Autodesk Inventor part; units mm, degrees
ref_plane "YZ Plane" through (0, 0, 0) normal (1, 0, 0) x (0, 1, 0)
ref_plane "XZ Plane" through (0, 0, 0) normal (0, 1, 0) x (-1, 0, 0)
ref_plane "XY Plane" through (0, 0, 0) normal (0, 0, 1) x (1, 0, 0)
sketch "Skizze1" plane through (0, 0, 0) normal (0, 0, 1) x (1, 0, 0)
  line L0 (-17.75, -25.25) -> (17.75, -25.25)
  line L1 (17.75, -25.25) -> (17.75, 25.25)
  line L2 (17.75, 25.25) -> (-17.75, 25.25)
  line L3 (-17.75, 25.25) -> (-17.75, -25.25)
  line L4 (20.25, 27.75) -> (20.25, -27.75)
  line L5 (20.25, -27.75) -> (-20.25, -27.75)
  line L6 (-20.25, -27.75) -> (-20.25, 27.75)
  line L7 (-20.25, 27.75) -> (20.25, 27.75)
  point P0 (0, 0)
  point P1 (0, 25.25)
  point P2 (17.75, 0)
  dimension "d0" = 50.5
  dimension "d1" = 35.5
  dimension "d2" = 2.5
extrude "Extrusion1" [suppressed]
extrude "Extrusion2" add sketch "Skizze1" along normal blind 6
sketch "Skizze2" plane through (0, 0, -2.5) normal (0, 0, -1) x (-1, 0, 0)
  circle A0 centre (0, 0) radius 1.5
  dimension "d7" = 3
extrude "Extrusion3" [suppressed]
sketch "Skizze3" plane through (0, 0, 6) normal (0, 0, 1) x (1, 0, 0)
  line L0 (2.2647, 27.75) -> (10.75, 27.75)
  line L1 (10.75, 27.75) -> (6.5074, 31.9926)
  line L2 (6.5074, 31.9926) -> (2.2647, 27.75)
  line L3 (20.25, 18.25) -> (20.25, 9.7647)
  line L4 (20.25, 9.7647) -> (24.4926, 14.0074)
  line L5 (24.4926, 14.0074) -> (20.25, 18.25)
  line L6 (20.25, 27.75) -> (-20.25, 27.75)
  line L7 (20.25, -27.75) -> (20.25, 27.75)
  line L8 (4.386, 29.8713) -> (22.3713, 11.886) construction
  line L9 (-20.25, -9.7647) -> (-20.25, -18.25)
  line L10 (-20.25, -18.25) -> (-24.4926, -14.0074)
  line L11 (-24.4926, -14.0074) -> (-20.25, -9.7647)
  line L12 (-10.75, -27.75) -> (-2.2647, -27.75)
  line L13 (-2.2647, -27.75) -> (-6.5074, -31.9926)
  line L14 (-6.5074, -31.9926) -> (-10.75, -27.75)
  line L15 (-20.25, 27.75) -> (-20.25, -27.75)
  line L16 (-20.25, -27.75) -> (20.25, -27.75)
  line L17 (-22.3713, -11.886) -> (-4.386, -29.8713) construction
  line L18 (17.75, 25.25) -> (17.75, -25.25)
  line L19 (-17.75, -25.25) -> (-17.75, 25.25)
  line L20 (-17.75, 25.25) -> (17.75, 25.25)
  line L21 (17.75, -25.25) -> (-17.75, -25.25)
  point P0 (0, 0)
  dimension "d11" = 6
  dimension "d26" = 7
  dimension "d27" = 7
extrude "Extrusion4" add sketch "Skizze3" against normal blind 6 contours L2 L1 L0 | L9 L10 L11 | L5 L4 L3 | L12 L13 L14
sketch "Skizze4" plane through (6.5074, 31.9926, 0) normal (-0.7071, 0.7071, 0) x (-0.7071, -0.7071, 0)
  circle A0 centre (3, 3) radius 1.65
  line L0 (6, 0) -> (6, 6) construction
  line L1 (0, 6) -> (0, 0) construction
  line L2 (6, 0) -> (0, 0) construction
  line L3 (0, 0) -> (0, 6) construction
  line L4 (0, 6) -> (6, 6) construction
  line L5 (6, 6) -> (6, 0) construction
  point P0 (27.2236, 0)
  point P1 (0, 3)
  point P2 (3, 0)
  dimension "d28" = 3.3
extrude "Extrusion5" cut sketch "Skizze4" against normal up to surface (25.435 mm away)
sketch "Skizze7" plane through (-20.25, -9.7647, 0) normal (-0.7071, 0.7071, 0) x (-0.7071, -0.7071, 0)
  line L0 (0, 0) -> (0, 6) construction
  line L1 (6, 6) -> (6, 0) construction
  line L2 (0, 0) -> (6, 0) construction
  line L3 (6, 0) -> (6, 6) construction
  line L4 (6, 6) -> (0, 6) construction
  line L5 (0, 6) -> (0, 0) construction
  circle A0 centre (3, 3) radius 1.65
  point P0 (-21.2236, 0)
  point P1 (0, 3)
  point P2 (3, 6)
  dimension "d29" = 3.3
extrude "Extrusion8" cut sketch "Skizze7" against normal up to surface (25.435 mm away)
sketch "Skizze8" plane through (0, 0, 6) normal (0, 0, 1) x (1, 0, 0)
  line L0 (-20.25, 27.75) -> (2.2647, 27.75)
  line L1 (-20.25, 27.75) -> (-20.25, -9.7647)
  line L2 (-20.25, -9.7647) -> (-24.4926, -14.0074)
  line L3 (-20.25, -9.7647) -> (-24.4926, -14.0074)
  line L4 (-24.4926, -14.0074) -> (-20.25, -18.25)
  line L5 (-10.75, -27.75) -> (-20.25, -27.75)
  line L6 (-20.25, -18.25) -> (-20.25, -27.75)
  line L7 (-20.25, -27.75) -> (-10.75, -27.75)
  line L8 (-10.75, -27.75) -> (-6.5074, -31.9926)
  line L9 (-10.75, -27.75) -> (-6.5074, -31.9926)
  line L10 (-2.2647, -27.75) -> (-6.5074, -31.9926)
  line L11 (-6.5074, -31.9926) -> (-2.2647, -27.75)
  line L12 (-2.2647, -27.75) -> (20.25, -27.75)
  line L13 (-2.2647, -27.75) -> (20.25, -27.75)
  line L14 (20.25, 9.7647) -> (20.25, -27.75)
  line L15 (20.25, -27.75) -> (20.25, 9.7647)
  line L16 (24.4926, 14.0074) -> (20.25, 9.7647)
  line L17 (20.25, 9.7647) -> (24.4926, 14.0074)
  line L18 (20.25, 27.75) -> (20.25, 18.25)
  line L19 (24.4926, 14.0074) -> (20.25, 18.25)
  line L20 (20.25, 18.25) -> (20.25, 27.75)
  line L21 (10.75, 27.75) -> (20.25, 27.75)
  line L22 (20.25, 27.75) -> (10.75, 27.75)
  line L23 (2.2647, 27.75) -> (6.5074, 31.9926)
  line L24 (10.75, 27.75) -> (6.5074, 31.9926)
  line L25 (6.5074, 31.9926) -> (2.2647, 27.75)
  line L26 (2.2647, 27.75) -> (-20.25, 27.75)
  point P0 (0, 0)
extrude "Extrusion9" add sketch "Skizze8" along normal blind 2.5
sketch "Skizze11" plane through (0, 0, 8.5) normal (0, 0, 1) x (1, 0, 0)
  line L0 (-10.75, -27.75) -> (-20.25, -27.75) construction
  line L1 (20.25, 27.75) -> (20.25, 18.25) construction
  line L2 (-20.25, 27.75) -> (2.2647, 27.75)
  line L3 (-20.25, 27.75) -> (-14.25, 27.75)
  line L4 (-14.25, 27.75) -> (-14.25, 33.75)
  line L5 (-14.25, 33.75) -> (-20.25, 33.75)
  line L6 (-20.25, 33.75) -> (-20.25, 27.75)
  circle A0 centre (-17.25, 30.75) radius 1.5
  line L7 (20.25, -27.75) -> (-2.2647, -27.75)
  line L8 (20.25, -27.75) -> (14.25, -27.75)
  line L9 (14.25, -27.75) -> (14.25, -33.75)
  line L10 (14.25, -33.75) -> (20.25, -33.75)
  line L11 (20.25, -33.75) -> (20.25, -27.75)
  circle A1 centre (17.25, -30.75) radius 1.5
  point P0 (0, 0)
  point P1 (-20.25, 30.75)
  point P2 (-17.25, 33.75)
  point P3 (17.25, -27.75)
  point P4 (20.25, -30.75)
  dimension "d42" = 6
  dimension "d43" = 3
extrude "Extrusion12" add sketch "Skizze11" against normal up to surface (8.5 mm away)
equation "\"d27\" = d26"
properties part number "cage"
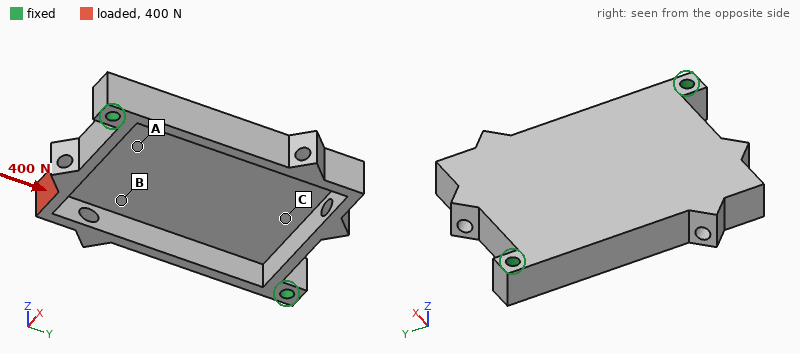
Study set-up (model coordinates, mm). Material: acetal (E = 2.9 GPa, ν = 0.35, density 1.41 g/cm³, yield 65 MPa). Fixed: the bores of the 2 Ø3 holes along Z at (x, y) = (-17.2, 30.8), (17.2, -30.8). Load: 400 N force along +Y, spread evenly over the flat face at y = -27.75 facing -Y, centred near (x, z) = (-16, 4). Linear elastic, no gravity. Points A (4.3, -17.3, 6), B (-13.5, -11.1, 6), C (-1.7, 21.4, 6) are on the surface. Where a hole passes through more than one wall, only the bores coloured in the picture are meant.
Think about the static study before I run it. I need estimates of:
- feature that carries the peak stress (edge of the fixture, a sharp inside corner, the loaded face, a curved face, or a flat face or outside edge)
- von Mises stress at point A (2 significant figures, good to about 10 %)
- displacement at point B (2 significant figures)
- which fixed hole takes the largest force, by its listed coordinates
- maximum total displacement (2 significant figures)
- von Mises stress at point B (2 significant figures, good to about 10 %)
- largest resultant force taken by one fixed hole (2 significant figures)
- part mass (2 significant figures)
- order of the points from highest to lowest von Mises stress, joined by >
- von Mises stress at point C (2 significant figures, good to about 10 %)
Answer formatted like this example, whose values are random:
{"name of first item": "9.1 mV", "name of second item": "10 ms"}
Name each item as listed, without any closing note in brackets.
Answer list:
{"feature that carries the peak stress": "a curved face", "von Mises stress at point A": "3.9 MPa", "displacement at point B": "0.11 mm", "which fixed hole takes the largest force, by its listed coordinates": "(-17.2, 30.8)", "maximum total displacement": "0.51 mm", "von Mises stress at point B": "7.2 MPa", "largest resultant force taken by one fixed hole": "310 N", "part mass": "13 g", "order of the points from highest to lowest von Mises stress, joined by >": "B > A > C", "von Mises stress at point C": "2.2 MPa"}
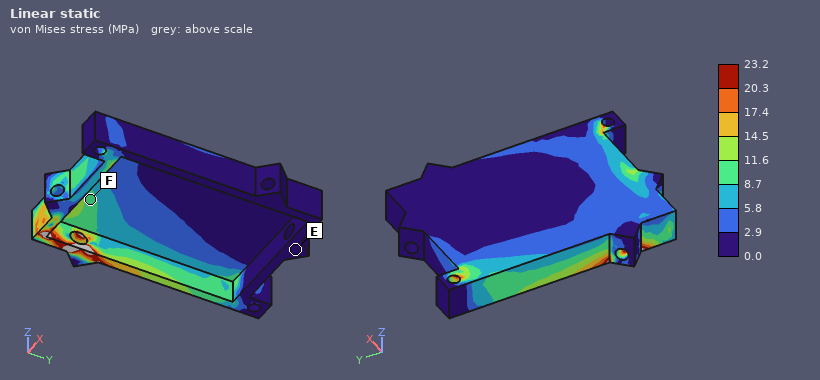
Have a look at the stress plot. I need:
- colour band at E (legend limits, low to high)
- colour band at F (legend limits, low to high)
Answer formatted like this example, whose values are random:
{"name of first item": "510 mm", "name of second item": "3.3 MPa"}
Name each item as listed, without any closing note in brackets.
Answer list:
{"colour band at E": "0.0 to 2.9 MPa", "colour band at F": "8.7 to 11.6 MPa"}
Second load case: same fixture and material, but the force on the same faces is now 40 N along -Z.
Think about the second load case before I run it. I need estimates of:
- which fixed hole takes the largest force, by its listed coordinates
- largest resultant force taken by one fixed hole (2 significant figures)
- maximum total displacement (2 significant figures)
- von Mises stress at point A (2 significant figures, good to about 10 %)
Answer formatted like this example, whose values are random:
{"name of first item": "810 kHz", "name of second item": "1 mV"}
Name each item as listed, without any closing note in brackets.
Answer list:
{"which fixed hole takes the largest force, by its listed coordinates": "(17.2, -30.8)", "largest resultant force taken by one fixed hole": "66 N", "maximum total displacement": "0.83 mm", "von Mises stress at point A": "2.7 MPa"}
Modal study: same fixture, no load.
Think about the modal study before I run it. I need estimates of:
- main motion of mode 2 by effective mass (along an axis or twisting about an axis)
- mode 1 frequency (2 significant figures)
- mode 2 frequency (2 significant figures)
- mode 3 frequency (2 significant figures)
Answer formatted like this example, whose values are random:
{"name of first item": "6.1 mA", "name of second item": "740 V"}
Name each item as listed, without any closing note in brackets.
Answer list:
{"main motion of mode 2 by effective mass": "along Z", "mode 1 frequency": "860 Hz", "mode 2 frequency": "1000 Hz", "mode 3 frequency": "2100 Hz"}
